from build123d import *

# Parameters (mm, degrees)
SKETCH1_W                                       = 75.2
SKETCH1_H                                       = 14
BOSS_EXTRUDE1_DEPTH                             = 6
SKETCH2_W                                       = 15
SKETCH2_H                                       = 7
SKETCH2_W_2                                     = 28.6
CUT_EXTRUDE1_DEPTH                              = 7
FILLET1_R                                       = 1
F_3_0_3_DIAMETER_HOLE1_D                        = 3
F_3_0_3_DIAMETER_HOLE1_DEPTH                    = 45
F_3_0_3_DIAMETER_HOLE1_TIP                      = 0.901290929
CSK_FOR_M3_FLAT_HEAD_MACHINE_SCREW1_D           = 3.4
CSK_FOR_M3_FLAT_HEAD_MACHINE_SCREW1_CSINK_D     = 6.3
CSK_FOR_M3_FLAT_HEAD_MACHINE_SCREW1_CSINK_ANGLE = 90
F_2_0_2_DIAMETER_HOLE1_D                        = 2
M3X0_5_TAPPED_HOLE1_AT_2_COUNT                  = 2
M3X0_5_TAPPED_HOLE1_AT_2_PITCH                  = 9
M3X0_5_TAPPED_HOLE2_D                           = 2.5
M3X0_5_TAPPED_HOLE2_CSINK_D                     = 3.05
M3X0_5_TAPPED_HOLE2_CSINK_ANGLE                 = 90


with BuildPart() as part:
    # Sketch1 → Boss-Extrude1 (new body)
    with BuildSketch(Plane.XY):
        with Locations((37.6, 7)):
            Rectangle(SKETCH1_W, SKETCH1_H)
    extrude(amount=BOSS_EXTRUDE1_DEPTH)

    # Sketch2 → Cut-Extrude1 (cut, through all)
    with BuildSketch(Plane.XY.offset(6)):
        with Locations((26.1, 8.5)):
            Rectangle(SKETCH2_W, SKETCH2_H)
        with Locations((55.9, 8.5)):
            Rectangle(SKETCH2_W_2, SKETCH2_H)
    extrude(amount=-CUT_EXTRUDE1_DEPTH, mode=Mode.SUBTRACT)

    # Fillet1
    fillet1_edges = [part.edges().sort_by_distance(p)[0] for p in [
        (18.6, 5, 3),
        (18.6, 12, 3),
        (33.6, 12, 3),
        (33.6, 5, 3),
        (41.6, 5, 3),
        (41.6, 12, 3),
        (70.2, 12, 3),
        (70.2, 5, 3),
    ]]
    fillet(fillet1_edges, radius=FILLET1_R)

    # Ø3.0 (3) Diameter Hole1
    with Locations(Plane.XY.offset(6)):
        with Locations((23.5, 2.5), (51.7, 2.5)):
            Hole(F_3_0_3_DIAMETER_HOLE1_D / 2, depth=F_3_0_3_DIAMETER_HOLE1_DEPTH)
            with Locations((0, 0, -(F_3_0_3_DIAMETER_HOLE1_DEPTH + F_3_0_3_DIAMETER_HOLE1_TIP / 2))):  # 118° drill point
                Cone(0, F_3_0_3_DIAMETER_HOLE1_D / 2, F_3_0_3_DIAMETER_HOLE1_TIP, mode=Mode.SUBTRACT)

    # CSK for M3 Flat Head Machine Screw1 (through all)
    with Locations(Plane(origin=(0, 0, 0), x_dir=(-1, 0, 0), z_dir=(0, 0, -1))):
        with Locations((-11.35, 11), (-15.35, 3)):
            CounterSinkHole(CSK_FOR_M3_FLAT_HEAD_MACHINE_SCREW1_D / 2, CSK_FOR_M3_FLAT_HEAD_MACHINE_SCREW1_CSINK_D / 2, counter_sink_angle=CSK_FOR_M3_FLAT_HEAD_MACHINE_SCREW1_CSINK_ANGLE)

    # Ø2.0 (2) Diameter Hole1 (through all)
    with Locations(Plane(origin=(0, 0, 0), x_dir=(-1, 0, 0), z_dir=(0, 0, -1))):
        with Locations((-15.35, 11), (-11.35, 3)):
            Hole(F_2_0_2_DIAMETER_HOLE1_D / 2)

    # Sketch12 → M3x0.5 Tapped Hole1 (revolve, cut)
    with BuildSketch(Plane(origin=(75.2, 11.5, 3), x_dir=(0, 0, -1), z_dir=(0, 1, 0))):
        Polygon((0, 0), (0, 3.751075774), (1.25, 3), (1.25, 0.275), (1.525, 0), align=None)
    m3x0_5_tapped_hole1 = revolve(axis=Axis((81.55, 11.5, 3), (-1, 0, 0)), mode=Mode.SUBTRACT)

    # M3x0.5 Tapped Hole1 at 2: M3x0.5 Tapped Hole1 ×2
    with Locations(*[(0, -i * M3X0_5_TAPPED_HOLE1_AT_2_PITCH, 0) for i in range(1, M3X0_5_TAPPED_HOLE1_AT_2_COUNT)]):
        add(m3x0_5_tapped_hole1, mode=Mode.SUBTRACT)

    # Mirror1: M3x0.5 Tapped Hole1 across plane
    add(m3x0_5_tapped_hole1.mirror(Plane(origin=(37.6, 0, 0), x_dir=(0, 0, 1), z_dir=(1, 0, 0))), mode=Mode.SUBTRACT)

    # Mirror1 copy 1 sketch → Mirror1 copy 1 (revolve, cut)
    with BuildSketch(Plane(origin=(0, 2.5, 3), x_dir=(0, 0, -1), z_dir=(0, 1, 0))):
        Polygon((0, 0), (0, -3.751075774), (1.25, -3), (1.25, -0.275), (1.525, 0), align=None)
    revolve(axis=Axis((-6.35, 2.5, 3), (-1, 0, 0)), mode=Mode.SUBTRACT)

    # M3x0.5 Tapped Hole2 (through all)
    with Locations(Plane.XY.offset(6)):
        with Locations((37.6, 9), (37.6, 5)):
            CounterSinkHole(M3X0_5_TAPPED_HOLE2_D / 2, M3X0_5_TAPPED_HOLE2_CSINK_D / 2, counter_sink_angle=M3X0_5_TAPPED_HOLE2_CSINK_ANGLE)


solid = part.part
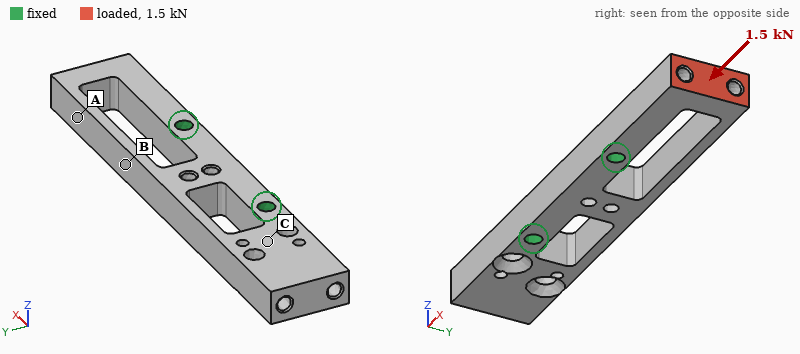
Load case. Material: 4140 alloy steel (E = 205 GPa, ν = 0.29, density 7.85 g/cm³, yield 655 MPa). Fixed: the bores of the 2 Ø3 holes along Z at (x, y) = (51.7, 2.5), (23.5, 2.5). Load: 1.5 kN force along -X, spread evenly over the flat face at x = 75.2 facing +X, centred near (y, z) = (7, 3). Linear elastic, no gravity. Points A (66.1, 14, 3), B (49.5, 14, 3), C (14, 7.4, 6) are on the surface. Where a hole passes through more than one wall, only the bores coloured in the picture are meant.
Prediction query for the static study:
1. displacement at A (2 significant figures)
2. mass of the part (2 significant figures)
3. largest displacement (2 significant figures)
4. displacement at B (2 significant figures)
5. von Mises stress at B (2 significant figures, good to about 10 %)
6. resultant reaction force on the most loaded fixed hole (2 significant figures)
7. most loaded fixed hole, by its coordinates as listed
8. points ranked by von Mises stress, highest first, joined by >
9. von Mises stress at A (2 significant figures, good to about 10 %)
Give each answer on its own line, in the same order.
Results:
18 µm
32 g
23 µm
13 µm
37 MPa
1.2 kN
(51.7, 2.5)
A > B > C
53 MPa
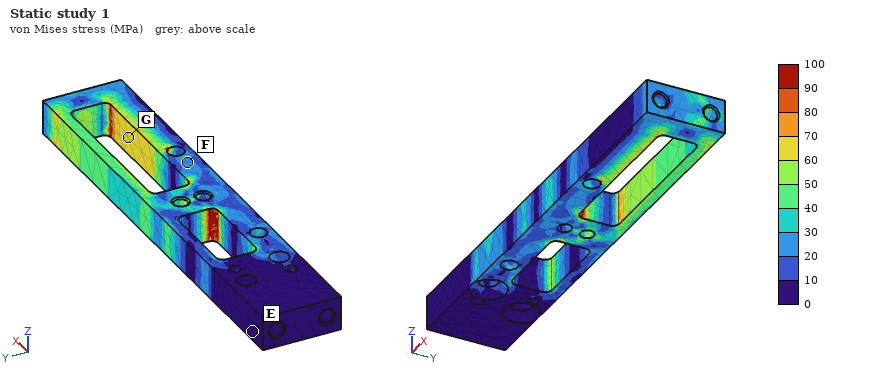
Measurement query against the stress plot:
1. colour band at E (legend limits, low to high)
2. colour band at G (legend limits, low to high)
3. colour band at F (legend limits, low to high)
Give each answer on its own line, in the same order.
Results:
0 to 10 MPa
60 to 70 MPa
20 to 30 MPa
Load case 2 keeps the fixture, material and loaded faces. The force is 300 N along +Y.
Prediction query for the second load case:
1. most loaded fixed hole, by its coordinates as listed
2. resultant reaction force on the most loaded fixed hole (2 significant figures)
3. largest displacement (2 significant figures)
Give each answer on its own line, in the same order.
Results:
(51.7, 2.5)
470 N
35 µm
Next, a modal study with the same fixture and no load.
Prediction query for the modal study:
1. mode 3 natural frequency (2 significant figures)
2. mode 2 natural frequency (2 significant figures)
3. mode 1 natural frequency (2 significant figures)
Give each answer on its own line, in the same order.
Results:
6600 Hz
5600 Hz
5500 Hz
